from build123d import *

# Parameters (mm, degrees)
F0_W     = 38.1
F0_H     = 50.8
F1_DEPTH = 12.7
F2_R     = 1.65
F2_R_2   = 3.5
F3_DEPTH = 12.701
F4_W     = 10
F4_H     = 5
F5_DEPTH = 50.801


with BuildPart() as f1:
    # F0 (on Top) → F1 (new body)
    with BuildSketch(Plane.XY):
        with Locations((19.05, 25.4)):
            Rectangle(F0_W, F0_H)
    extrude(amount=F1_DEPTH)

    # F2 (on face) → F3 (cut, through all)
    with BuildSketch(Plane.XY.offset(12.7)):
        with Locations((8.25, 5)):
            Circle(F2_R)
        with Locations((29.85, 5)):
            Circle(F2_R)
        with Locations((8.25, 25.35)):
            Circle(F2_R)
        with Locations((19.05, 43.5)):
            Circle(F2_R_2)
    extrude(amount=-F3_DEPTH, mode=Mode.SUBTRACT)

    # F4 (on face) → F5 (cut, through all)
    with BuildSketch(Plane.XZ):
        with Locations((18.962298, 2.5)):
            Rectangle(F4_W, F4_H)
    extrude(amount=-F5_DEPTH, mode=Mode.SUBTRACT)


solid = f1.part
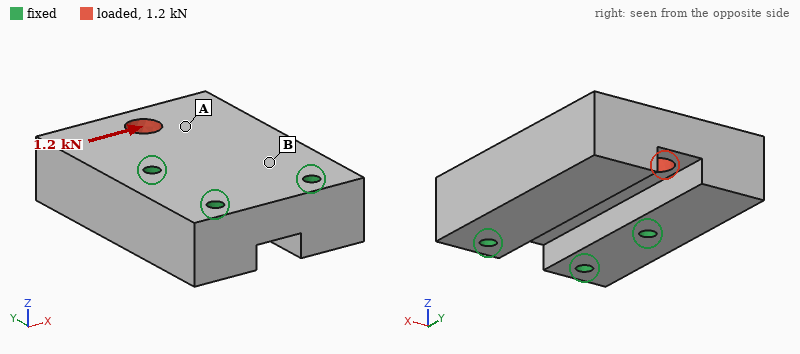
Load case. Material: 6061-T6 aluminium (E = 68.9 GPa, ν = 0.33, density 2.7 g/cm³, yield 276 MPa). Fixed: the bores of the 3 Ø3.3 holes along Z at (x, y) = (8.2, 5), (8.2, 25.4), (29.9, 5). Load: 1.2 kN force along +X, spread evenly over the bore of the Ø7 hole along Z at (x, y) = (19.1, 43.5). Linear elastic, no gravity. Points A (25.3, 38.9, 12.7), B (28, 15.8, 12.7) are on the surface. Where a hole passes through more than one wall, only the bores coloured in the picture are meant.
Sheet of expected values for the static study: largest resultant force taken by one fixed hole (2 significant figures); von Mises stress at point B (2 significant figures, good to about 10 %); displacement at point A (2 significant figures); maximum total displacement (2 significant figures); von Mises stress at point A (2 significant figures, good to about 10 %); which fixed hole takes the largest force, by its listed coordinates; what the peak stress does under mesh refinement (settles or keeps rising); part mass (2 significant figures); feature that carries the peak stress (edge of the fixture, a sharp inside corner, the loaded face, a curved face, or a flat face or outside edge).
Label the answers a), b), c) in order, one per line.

a) 1.4 kN
b) 4.1 MPa
c) 4.8 µm
d) 8.5 µm
e) 7.7 MPa
f) (8.2, 25.4)
g) keeps rising
h) 58 g
i) edge of the fixture
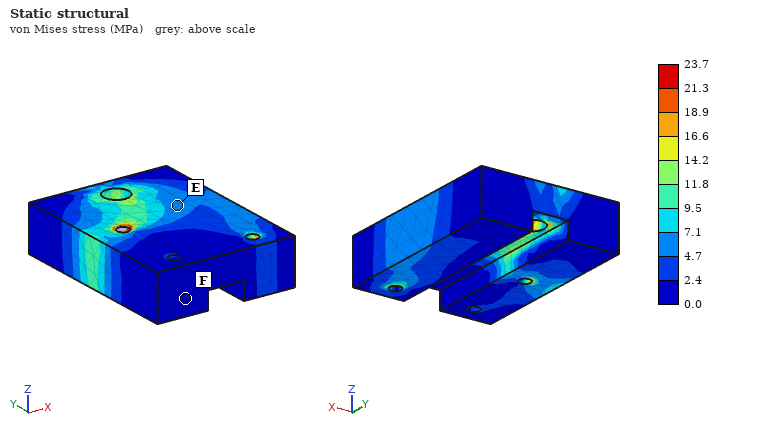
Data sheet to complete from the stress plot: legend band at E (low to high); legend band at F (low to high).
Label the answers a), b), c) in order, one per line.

a) 4.7 to 7.1 MPa
b) 0.0 to 2.4 MPa
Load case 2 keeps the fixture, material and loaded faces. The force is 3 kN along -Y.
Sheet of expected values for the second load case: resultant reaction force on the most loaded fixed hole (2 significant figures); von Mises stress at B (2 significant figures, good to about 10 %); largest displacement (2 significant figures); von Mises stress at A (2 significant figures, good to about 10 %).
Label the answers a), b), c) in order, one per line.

a) 1.4 kN
b) 11 MPa
c) 13 µm
d) 20 MPa
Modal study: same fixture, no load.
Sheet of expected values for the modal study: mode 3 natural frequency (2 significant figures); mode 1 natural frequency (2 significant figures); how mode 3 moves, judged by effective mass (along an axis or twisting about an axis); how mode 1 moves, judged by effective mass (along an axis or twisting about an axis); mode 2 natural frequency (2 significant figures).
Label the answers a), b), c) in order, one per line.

a) 16 kHz
b) 7300 Hz
c) along X
d) along Z
e) 14 kHz
